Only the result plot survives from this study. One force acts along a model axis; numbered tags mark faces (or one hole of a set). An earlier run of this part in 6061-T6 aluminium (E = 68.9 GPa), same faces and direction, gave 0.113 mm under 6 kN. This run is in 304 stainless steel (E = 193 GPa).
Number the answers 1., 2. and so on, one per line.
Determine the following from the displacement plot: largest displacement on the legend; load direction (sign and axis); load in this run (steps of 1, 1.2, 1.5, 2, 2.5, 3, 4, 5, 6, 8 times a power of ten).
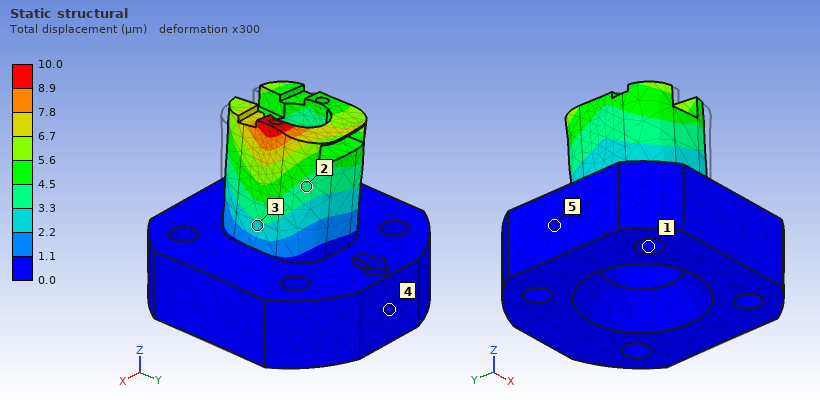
1. 10.0 µm
2. -X
3. 1.5 kN
